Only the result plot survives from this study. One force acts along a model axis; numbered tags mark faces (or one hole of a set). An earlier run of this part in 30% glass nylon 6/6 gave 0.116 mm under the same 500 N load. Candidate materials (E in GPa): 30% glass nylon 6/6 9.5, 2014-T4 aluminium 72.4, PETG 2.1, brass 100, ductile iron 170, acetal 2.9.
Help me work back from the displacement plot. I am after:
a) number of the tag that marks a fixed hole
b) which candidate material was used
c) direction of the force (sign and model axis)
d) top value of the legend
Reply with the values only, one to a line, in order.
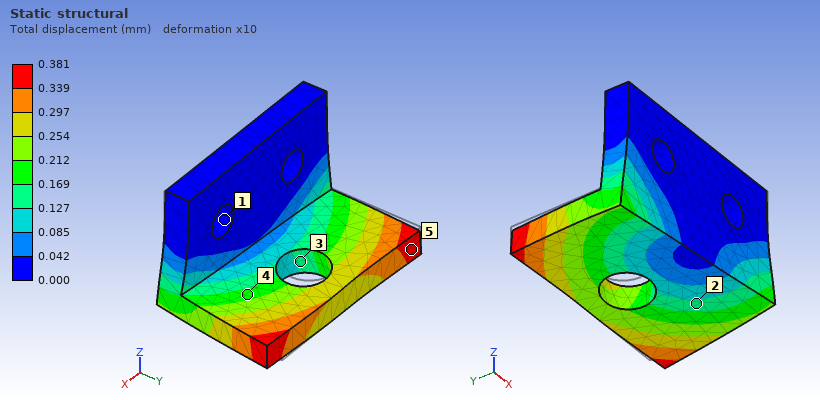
1
acetal
+X
0.381 mm
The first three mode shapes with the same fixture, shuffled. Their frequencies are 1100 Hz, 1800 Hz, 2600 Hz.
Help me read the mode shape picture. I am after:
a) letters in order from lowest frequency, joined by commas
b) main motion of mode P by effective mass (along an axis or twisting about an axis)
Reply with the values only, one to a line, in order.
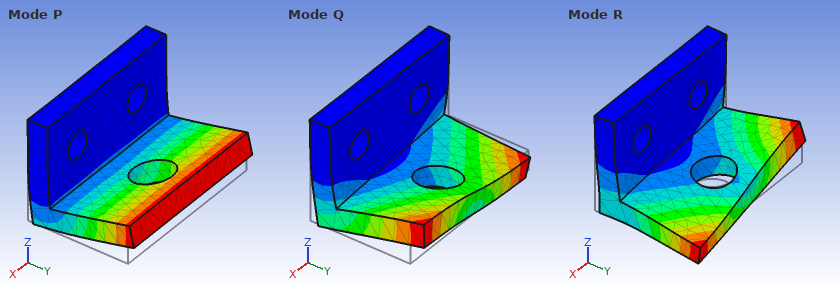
P, Q, R
along Z
